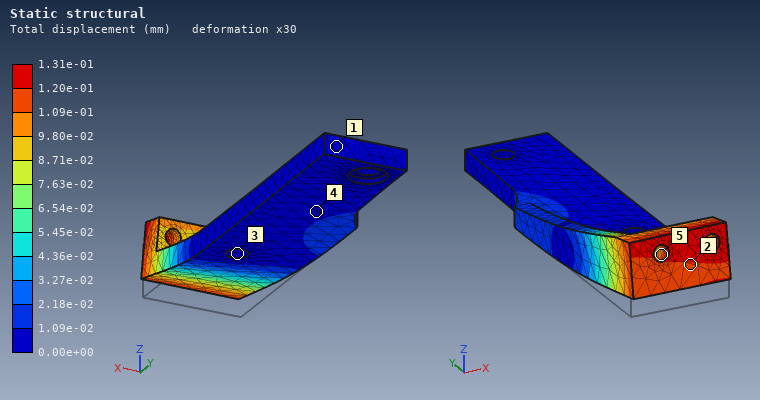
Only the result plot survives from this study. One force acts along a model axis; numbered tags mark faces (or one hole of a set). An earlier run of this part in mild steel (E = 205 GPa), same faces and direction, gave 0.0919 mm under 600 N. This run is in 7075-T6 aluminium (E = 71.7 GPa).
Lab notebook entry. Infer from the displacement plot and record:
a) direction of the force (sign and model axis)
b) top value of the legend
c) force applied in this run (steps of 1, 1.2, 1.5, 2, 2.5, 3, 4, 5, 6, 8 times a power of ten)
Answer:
+Z
1.31e-01 mm
300 N
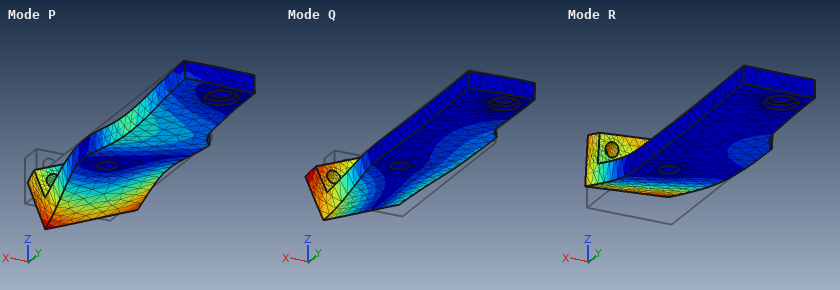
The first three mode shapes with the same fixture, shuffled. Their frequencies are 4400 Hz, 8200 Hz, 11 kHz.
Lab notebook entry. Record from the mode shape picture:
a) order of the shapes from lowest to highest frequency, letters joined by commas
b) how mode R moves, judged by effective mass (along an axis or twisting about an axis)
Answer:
R, Q, P
along Z
